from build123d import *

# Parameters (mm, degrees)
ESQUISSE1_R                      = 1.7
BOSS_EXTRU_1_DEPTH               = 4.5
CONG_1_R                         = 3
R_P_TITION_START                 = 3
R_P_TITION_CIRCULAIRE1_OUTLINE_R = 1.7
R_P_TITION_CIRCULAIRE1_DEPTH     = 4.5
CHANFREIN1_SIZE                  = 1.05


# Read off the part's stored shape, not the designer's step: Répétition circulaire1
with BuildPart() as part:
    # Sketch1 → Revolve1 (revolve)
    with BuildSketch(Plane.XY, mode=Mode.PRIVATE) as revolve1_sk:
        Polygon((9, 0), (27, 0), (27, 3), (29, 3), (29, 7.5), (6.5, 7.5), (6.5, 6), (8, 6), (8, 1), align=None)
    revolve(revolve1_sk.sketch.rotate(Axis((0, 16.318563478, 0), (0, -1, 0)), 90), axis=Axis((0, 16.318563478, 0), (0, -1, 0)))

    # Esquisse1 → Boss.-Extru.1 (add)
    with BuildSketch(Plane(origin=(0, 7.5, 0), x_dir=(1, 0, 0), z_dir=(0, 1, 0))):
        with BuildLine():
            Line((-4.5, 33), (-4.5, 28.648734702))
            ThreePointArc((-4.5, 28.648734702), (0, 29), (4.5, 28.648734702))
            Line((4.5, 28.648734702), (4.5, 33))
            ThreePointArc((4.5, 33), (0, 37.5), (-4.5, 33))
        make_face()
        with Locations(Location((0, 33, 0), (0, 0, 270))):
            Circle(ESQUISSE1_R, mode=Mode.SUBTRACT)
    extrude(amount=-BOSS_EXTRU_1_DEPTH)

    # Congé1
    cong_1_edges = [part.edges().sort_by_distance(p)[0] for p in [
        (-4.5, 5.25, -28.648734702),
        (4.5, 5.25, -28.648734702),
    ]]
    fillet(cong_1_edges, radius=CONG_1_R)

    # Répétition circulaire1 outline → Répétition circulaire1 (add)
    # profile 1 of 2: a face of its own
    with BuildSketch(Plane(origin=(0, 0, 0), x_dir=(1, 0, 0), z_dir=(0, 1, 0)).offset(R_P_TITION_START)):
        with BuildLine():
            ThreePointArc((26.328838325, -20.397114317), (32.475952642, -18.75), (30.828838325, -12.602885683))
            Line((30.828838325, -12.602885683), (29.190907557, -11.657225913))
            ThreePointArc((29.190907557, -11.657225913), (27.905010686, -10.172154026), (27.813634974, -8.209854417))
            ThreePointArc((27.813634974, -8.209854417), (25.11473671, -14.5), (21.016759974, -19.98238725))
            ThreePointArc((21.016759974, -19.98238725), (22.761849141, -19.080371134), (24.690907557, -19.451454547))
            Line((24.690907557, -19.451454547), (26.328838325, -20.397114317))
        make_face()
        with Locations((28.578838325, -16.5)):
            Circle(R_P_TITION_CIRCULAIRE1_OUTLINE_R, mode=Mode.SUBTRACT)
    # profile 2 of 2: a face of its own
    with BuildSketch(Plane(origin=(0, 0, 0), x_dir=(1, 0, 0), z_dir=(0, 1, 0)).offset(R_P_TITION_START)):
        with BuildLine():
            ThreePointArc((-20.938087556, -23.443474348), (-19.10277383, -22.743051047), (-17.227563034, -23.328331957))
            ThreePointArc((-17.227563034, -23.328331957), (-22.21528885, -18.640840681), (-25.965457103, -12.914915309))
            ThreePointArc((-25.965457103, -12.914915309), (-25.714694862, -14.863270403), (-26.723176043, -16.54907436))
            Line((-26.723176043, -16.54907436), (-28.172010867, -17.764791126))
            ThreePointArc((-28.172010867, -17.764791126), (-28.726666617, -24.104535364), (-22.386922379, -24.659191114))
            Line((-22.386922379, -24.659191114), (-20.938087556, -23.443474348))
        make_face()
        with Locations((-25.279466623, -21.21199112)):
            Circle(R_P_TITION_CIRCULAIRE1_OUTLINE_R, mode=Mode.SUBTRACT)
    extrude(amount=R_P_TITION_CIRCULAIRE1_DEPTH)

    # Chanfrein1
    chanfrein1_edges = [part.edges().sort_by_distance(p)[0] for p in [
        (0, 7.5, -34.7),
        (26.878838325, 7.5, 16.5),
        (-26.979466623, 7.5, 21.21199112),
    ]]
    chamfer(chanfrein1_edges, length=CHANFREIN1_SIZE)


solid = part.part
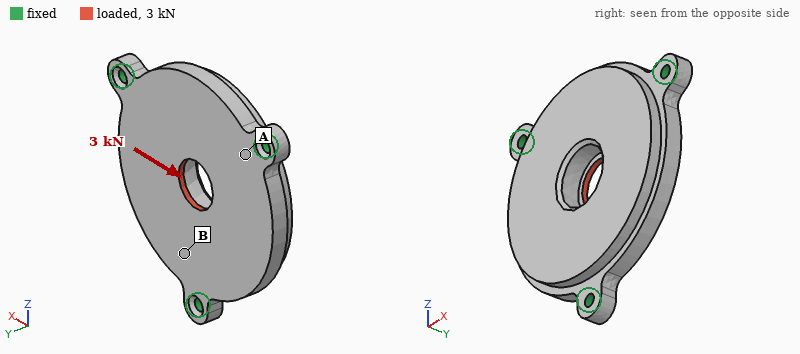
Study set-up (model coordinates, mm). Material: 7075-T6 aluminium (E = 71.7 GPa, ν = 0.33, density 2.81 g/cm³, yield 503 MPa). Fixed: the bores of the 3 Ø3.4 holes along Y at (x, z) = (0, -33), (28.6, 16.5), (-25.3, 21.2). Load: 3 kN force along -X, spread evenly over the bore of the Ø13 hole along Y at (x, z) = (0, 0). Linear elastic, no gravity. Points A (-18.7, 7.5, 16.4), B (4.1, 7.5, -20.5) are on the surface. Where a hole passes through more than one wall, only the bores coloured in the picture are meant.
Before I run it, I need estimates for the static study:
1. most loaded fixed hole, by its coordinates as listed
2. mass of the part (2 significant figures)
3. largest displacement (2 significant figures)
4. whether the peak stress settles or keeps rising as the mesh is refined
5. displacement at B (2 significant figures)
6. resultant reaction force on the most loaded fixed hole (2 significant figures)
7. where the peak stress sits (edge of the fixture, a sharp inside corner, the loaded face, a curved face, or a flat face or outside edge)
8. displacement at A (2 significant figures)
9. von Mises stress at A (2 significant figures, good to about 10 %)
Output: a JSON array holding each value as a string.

["(28.6, 16.5)", "51 g", "18 µm", "keeps rising", "8.9 µm", "1.2 kN", "edge of the fixture", "4.8 µm", "22 MPa"]
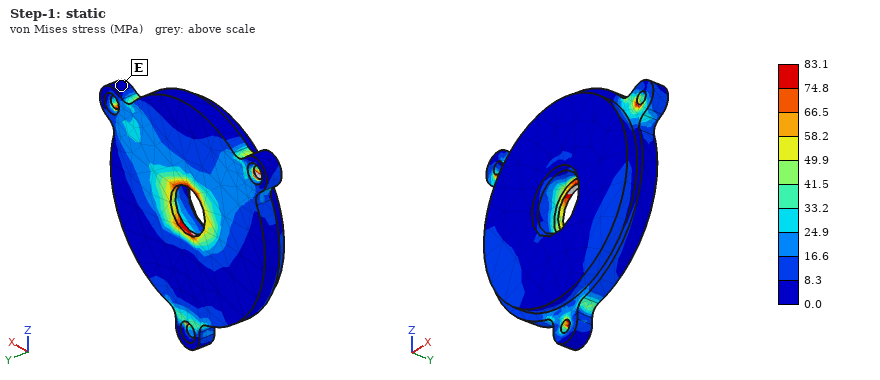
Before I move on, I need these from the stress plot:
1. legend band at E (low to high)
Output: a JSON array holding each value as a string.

["0.0 to 8.3 MPa"]
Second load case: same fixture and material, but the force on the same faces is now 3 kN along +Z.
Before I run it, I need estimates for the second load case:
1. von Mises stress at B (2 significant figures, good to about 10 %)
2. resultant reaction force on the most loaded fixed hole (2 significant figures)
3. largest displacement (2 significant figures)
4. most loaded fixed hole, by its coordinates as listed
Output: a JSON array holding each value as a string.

["23 MPa", "1.3 kN", "14 µm", "(0, -33)"]
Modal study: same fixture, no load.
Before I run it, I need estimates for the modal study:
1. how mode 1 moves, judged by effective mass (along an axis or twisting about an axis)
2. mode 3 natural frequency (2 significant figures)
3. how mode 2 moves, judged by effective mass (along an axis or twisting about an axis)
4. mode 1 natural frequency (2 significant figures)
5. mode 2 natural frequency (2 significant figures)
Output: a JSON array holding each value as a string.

["along Y", "8000 Hz", "along Y", "5800 Hz", "6800 Hz"]
